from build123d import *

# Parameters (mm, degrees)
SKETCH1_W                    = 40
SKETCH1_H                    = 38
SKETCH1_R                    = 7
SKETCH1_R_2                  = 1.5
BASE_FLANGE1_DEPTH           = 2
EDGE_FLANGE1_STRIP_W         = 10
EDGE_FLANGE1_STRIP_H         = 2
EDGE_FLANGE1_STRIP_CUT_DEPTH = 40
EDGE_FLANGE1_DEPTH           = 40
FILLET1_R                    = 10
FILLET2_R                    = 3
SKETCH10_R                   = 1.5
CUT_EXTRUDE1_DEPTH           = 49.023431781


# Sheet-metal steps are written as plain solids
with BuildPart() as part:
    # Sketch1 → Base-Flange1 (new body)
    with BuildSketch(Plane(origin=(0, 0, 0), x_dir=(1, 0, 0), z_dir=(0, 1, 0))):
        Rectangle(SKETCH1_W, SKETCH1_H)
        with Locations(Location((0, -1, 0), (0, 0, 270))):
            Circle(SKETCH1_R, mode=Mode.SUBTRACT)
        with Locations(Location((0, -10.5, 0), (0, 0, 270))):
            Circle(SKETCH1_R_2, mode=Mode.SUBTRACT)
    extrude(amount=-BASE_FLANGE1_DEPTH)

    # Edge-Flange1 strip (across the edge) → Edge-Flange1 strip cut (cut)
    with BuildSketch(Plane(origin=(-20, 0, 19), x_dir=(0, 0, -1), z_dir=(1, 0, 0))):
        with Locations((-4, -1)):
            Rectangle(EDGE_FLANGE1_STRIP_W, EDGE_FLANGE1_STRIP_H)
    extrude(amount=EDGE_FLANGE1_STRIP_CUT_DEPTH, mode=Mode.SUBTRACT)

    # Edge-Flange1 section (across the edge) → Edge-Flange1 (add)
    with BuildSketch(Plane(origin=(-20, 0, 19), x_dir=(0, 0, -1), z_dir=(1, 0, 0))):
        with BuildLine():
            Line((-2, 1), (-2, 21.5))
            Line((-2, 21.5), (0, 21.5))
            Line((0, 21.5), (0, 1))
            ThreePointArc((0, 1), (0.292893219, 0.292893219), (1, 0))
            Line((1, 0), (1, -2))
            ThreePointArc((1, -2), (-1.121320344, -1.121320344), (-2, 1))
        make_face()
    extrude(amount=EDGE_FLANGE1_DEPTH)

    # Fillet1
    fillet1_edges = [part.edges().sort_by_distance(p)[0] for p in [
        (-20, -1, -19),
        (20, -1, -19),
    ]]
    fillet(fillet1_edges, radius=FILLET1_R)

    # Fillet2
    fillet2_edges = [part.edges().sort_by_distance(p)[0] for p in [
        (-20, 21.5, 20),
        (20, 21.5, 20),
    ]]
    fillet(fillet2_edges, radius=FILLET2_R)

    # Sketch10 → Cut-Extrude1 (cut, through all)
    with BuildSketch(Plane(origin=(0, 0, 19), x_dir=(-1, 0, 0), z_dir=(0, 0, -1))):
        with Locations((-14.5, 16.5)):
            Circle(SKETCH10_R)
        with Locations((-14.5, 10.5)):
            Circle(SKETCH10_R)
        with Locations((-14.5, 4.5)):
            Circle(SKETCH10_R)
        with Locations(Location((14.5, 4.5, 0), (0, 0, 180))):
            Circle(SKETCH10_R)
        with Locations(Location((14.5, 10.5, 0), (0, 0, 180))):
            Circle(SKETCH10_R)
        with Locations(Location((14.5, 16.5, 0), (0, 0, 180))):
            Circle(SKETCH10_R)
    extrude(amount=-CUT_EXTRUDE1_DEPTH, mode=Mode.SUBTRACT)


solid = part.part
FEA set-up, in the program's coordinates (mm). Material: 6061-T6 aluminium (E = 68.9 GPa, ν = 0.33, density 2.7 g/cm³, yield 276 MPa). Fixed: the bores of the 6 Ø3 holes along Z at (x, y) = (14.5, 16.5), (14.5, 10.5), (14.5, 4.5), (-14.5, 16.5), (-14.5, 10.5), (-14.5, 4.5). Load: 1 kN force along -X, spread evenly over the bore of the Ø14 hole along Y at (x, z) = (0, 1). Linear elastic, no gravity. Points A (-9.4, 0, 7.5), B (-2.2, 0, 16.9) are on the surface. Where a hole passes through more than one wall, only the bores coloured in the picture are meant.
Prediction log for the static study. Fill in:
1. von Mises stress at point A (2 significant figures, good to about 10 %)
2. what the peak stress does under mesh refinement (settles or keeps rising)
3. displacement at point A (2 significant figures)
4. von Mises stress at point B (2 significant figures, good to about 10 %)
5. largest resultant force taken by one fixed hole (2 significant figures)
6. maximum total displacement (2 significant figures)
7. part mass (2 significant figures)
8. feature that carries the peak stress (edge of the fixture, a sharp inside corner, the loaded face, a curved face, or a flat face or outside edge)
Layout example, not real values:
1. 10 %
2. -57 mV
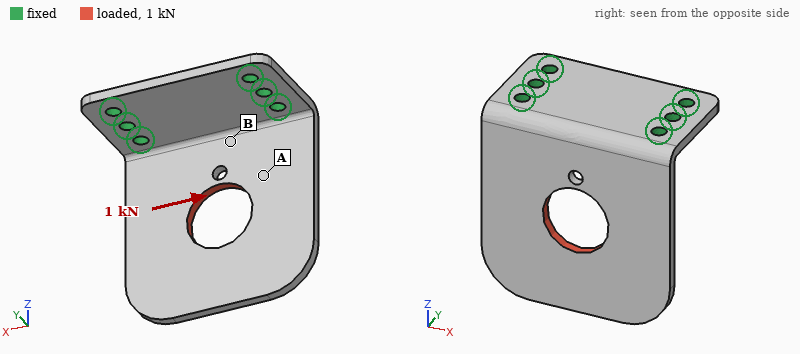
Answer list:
1. 43 MPa
2. keeps rising
3. 0.069 mm
4. 79 MPa
5. 830 N
6. 0.18 mm
7. 12 g
8. edge of the fixture
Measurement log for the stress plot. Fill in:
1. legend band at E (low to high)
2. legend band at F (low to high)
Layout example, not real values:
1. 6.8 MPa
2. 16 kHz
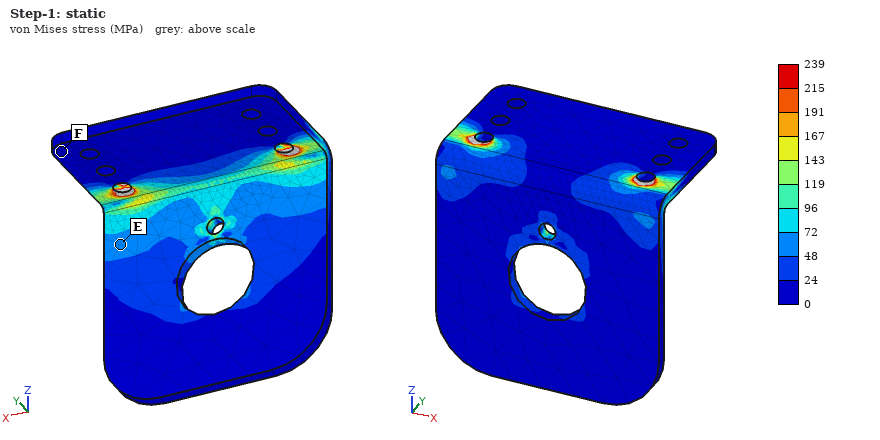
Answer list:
1. 48 to 72 MPa
2. 0 to 24 MPa
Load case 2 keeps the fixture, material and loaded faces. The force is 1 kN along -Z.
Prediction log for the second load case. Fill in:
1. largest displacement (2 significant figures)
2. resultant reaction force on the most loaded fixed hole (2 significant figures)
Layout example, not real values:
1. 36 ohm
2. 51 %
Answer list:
1. 0.33 mm
2. 610 N
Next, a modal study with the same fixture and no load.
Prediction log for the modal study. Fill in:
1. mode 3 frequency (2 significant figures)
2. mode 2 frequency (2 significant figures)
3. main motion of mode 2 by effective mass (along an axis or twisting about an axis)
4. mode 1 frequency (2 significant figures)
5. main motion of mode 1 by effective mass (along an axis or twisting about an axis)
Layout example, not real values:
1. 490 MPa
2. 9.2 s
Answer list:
1. 5400 Hz
2. 2400 Hz
3. twisting about Z
4. 930 Hz
5. along Y
